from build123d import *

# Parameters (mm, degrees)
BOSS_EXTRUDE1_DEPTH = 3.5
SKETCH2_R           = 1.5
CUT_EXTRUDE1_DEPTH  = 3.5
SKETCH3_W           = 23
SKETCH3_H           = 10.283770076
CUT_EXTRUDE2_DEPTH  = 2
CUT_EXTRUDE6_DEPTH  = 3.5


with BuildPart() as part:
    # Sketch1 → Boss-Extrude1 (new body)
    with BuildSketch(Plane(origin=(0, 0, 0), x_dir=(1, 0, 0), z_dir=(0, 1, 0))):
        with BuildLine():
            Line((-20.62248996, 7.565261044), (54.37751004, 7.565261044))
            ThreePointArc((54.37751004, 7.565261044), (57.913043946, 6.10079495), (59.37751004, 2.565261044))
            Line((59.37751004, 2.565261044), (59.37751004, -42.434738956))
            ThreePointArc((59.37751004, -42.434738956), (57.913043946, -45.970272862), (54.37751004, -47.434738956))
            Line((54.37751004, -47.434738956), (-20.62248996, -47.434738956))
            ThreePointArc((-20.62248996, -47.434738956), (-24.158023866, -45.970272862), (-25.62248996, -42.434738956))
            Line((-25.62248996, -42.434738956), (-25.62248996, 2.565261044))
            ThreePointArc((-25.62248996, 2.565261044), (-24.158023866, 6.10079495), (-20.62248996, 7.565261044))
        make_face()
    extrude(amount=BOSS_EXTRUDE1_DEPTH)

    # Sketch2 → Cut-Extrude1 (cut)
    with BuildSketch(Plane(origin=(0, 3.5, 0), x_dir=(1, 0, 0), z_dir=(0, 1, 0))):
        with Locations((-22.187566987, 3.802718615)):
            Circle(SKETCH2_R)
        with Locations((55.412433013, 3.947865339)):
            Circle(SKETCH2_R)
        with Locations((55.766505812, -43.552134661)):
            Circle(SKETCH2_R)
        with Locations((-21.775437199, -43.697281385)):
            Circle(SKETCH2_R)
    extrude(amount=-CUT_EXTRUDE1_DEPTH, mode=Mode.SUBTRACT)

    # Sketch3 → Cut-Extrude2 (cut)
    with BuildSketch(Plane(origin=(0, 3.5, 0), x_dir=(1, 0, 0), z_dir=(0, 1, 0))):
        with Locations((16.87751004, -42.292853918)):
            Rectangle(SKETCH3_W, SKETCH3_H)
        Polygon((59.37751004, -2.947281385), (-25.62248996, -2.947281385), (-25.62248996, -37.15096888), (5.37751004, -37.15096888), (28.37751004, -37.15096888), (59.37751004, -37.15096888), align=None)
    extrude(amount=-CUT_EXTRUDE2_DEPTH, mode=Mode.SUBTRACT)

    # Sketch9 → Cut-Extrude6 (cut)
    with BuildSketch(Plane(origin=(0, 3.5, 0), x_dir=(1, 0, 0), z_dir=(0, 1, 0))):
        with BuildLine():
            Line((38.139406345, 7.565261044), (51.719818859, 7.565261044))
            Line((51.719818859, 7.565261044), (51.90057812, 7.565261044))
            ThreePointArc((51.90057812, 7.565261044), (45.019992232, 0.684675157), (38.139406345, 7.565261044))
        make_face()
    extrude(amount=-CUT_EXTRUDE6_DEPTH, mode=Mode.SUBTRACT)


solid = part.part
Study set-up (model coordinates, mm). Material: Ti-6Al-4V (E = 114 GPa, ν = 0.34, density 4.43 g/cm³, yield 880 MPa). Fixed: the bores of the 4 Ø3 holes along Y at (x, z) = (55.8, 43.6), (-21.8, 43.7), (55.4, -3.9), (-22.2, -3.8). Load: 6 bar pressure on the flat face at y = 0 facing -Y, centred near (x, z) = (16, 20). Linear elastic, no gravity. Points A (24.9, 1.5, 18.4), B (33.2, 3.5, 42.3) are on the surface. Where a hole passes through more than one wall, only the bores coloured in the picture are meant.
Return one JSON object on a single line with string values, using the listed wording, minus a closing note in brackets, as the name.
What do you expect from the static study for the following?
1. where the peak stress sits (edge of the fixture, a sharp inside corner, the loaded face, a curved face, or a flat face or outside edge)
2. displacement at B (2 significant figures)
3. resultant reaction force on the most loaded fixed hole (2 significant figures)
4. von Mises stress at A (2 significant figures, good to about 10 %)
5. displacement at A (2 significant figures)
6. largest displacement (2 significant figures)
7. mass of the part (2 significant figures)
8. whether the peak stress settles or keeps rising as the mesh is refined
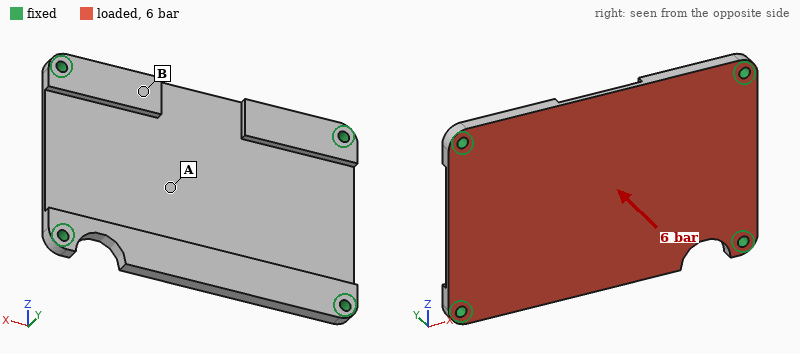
{"where the peak stress sits": "edge of the fixture", "displacement at B": "0.27 mm", "resultant reaction force on the most loaded fixed hole": "2.0 kN", "von Mises stress at A": "120 MPa", "displacement at A": "0.52 mm", "largest displacement": "0.56 mm", "mass of the part": "43 g", "whether the peak stress settles or keeps rising as the mesh is refined": "keeps rising"}
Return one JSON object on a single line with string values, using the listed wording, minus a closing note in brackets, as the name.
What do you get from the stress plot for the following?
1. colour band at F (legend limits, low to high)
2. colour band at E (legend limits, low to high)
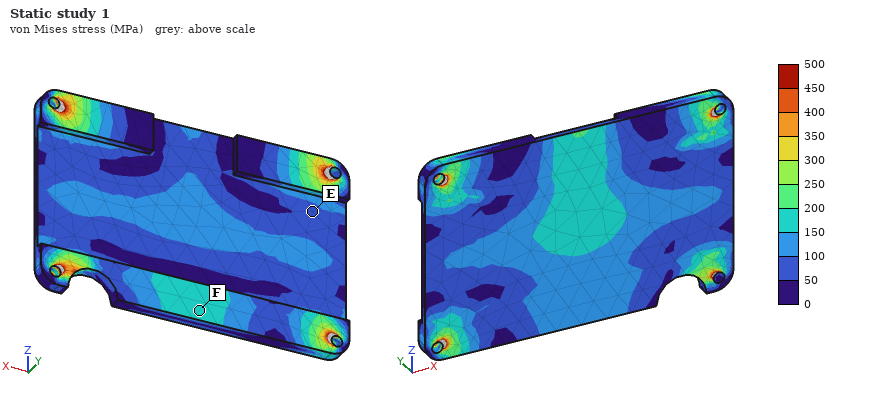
{"colour band at F": "150 to 200 MPa", "colour band at E": "50 to 100 MPa"}
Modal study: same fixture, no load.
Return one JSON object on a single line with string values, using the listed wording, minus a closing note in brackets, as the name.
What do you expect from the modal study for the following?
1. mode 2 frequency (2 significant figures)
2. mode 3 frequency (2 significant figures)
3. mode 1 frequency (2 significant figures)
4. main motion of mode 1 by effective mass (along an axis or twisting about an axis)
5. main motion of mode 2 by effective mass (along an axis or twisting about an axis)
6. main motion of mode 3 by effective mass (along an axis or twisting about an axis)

{"mode 2 frequency": "3100 Hz", "mode 3 frequency": "4700 Hz", "mode 1 frequency": "2300 Hz", "main motion of mode 1 by effective mass": "along Y", "main motion of mode 2 by effective mass": "twisting about X", "main motion of mode 3 by effective mass": "twisting about Z"}
